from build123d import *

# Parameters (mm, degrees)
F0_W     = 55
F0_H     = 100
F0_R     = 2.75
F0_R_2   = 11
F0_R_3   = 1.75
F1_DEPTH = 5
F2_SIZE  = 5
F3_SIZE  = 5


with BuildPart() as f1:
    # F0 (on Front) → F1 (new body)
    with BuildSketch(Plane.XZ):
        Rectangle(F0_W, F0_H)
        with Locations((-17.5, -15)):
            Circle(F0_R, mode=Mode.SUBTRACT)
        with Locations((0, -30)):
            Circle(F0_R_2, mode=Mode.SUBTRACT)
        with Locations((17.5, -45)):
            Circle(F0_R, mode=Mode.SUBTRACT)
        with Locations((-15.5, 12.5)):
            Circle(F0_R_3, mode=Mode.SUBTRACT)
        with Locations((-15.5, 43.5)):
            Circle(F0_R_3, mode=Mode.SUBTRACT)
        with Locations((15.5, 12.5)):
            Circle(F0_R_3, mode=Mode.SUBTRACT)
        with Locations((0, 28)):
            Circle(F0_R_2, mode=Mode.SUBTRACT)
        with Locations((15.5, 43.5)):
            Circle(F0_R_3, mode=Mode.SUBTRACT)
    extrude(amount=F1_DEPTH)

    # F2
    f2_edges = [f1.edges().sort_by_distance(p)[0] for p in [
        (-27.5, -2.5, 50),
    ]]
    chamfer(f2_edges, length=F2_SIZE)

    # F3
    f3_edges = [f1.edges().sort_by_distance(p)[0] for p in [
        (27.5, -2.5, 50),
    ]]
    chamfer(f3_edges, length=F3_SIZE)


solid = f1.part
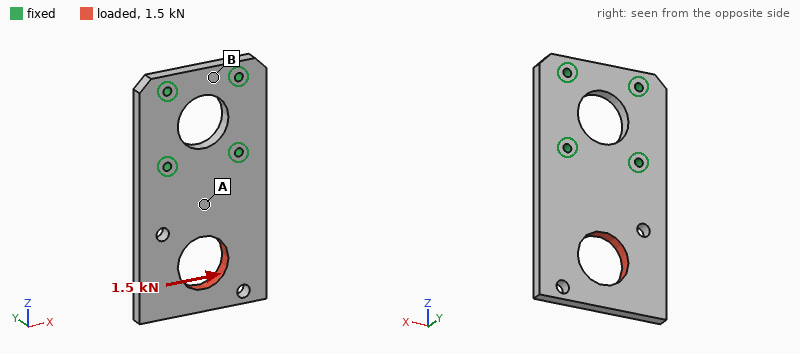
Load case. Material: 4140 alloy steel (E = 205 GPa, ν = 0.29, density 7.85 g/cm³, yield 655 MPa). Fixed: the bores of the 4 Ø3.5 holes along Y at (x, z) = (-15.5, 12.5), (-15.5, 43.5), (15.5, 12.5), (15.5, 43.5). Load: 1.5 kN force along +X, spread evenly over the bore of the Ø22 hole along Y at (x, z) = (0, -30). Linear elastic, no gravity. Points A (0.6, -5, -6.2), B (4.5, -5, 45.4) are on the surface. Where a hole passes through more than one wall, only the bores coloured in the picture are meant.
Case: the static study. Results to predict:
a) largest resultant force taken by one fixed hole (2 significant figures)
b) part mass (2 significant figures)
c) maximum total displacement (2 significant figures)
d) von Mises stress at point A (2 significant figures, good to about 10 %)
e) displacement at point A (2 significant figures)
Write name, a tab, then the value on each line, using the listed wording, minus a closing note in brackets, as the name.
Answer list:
largest resultant force taken by one fixed hole	1.7 kN
part mass	180 g
maximum total displacement	15 µm
von Mises stress at point A	20 MPa
displacement at point A	3.1 µm
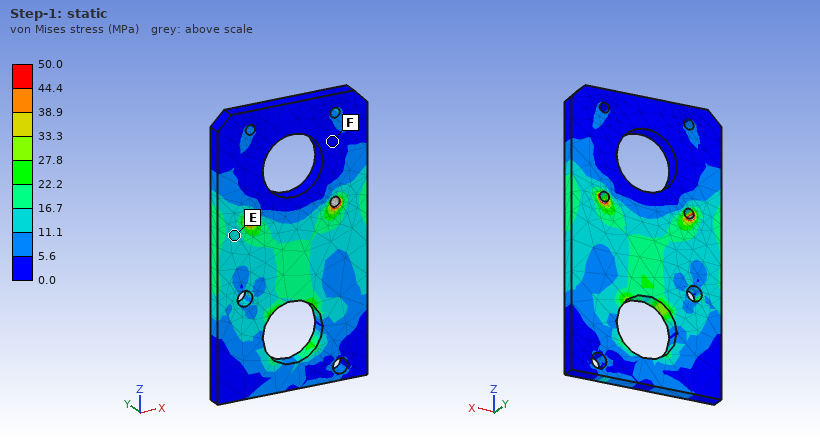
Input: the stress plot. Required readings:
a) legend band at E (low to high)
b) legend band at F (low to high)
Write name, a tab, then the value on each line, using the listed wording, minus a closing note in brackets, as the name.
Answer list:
legend band at E	11.1 to 16.7 MPa
legend band at F	0.0 to 5.6 MPa
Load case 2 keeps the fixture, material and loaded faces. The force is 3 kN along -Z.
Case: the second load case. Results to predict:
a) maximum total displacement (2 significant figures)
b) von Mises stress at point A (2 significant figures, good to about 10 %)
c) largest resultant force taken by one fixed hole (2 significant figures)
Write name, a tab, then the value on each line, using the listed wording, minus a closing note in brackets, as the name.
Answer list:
maximum total displacement	6.0 µm
von Mises stress at point A	8.6 MPa
largest resultant force taken by one fixed hole	1.3 kN
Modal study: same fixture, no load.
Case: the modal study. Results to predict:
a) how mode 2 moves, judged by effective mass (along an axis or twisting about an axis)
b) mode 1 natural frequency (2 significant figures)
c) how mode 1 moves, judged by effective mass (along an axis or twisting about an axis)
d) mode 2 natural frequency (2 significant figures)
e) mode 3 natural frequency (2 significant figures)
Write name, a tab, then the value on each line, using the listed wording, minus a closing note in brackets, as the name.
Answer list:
how mode 2 moves, judged by effective mass	twisting about Z
mode 1 natural frequency	1100 Hz
how mode 1 moves, judged by effective mass	along Y
mode 2 natural frequency	2600 Hz
mode 3 natural frequency	5600 Hz
